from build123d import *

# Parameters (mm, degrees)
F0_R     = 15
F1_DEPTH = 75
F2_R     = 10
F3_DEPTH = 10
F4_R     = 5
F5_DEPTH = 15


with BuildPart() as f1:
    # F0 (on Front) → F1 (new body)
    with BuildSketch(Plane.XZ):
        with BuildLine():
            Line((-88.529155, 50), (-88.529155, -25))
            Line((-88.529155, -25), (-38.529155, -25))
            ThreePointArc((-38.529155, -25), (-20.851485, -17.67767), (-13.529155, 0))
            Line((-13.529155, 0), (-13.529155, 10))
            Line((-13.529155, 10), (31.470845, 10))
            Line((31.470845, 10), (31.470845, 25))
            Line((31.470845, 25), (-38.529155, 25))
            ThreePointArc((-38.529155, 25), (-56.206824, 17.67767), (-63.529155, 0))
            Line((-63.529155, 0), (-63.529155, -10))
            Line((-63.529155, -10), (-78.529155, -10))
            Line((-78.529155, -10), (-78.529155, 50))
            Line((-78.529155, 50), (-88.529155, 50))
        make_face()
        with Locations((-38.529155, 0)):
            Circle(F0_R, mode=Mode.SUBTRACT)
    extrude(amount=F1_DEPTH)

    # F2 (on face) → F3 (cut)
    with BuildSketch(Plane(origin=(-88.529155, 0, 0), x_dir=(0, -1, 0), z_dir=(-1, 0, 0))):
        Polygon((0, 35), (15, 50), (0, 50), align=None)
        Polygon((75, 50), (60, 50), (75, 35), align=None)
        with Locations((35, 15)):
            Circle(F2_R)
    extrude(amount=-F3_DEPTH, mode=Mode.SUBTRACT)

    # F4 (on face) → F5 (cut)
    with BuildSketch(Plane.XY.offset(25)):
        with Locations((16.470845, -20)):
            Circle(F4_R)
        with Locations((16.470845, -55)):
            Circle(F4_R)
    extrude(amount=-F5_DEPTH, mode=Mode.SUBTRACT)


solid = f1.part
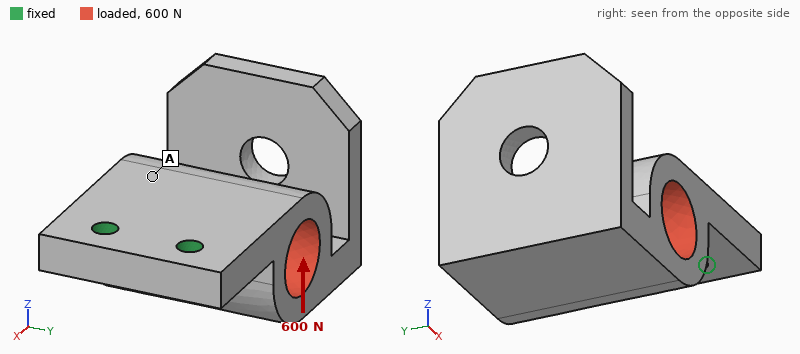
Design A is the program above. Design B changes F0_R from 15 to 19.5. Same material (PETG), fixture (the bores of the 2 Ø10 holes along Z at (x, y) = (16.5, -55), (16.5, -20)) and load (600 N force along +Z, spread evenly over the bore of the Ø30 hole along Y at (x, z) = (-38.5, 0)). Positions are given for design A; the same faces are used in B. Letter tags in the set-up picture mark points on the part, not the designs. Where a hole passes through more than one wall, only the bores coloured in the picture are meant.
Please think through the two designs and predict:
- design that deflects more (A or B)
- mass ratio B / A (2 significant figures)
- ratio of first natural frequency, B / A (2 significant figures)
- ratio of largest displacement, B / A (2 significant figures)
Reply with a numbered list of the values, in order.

1. B
2. 0.84
3. 0.90
4. 1.3
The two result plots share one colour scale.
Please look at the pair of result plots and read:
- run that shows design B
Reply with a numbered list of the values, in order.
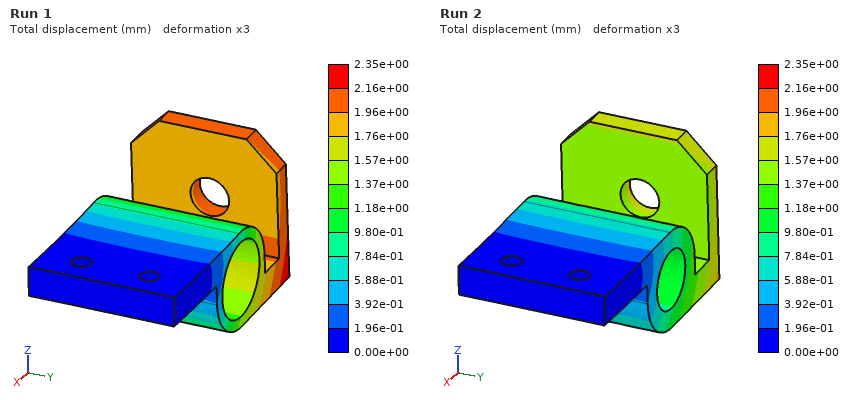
1. Run 1
